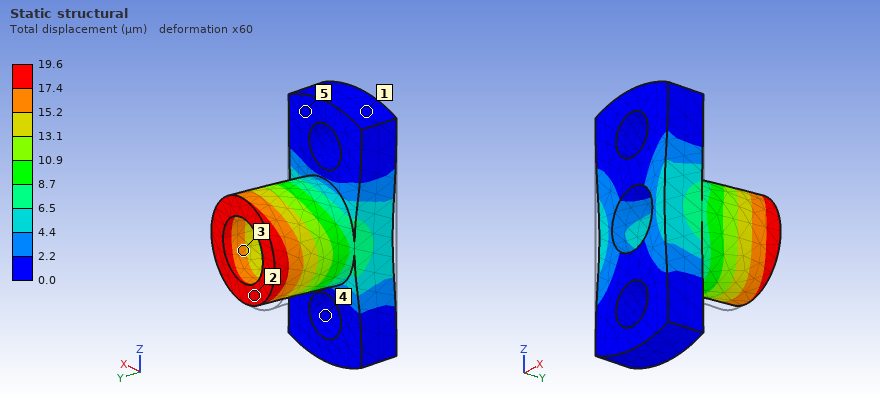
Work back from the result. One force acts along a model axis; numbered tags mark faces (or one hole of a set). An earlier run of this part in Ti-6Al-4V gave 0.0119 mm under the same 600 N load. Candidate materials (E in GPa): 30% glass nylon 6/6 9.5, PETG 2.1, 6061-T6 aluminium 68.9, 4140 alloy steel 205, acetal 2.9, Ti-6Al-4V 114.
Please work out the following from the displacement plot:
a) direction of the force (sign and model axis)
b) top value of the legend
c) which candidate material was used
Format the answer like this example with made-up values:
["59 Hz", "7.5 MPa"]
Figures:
["+X", "19.6 µm", "6061-T6 aluminium"]
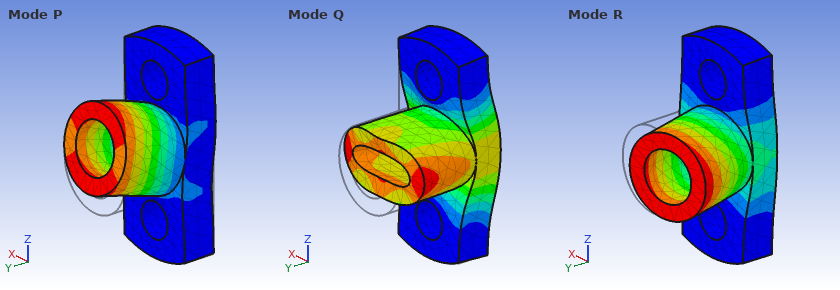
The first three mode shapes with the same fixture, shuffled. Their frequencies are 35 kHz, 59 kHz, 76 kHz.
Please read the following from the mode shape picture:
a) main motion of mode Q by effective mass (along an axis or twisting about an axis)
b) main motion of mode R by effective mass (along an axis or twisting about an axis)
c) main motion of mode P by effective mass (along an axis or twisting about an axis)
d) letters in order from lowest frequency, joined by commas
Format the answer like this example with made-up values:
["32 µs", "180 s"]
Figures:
["along Y", "along X", "along Z", "R, P, Q"]
